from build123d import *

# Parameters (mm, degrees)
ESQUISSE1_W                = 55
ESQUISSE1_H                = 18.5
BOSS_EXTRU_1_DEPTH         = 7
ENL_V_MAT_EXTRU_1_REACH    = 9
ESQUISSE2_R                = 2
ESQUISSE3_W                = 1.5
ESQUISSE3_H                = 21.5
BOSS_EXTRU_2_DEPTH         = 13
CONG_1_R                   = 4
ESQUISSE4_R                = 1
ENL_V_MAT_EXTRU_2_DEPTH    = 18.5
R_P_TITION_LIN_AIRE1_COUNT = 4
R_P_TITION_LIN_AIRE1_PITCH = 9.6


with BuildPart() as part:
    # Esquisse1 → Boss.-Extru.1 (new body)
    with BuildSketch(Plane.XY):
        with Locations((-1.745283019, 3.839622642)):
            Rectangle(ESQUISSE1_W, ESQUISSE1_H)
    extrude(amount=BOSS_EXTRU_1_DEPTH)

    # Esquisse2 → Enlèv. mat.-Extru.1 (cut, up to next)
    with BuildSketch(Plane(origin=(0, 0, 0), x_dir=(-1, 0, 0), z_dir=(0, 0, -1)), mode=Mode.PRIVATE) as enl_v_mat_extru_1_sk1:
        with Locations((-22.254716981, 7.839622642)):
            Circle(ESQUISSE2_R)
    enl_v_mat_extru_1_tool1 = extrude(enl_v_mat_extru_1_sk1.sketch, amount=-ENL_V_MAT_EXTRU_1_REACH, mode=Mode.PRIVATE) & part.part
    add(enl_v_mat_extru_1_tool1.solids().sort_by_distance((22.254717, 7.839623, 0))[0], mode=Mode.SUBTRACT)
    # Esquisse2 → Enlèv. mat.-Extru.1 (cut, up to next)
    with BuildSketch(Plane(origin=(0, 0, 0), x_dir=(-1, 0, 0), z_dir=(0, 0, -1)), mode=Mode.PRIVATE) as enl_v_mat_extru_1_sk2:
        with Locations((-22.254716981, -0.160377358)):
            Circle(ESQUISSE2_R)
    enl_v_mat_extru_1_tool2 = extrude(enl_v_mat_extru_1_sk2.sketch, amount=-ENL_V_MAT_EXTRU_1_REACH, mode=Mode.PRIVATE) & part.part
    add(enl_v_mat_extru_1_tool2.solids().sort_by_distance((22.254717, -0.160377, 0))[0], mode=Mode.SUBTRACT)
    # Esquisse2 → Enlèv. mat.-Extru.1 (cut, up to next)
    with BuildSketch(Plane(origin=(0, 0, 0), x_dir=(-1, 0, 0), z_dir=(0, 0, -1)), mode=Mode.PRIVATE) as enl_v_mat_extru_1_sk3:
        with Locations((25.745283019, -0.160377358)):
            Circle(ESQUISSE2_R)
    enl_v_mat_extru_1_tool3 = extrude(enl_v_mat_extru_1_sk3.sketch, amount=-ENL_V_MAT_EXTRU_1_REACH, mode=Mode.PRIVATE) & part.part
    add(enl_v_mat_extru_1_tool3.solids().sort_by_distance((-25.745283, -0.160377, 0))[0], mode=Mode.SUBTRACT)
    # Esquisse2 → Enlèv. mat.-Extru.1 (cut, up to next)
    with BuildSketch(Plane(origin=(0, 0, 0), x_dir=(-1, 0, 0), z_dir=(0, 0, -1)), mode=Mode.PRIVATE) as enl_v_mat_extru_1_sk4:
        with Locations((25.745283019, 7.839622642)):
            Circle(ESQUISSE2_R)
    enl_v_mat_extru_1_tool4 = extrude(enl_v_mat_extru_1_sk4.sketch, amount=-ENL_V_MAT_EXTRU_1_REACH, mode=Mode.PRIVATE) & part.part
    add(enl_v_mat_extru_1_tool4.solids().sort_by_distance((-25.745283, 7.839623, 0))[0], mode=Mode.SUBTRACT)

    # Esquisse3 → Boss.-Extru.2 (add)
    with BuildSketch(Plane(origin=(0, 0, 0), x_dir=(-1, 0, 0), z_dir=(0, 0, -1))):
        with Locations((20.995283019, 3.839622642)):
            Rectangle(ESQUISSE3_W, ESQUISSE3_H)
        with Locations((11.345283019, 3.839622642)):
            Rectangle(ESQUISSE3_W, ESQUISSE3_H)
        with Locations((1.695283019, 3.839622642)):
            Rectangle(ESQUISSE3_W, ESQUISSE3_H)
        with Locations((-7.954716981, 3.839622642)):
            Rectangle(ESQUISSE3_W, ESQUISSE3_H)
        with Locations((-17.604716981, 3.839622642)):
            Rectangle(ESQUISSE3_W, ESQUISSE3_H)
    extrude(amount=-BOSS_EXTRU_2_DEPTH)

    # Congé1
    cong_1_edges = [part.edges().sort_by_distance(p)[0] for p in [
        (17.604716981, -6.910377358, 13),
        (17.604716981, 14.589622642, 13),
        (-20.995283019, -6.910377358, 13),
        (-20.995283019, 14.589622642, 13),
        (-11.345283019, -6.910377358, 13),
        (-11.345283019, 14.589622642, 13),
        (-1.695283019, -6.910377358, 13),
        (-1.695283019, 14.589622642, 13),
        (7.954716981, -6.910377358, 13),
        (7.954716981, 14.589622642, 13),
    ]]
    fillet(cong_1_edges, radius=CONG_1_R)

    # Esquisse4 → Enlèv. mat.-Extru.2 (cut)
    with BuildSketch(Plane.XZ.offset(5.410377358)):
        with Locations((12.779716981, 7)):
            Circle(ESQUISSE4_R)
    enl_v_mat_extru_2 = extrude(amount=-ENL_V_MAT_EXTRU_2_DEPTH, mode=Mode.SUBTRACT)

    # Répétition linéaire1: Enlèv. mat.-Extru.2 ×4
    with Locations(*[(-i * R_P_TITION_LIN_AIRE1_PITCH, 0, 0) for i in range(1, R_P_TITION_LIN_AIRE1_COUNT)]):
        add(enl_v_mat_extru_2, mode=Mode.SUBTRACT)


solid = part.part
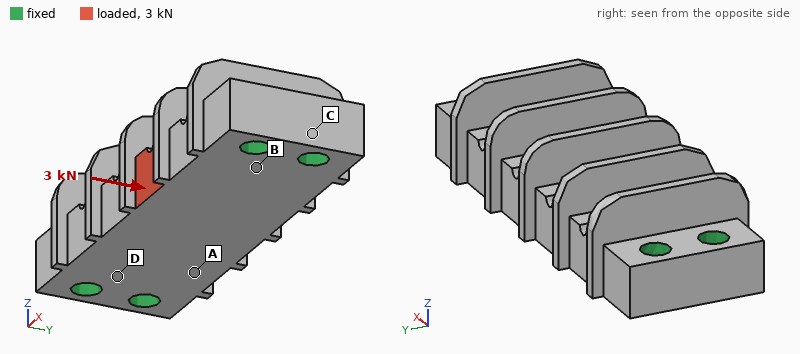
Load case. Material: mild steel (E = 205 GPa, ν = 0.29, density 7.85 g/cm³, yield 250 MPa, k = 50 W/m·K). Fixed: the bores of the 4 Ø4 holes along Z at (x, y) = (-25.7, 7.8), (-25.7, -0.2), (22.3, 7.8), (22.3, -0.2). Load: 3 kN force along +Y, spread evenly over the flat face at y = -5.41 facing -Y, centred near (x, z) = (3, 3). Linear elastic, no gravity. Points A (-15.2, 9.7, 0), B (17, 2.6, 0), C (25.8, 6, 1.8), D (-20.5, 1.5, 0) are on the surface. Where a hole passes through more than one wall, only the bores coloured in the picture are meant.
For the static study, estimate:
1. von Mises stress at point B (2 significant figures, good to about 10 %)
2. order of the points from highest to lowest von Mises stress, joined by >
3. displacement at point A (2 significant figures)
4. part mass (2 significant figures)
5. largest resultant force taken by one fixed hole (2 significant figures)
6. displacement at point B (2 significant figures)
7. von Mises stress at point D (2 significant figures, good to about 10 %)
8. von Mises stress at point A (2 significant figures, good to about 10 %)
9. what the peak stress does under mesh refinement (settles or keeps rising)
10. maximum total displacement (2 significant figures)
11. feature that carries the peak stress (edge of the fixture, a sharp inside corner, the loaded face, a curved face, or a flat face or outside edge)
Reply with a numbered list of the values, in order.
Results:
1. 42 MPa
2. B > D > A > C
3. 2.3 µm
4. 61 g
5. 1.7 kN
6. 1.2 µm
7. 24 MPa
8. 15 MPa
9. keeps rising
10. 7.2 µm
11. a sharp inside corner
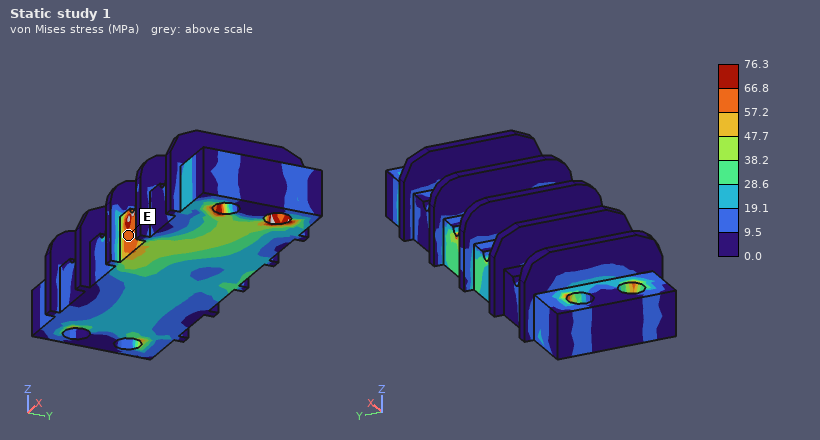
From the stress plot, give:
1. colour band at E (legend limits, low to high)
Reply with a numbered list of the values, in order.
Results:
1. 57.2 to 66.8 MPa
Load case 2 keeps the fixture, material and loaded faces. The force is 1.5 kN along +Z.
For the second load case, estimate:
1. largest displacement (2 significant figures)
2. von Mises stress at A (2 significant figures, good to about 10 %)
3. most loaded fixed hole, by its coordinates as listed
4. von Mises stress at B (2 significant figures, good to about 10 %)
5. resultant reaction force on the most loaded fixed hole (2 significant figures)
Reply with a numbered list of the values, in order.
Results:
1. 19 µm
2. 29 MPa
3. (22.3, -0.2)
4. 55 MPa
5. 1.0 kN
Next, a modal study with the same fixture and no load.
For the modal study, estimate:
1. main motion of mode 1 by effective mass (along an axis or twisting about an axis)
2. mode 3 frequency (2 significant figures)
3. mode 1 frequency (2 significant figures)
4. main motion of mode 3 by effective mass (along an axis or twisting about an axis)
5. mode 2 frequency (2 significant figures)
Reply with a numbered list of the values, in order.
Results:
1. along Z
2. 23 kHz
3. 14 kHz
4. along Y
5. 19 kHz
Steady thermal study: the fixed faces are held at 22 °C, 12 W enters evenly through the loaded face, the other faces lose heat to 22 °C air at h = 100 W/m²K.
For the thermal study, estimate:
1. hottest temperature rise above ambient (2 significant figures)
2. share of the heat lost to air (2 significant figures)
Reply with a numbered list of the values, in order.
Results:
1. 32 K
2. 25 %
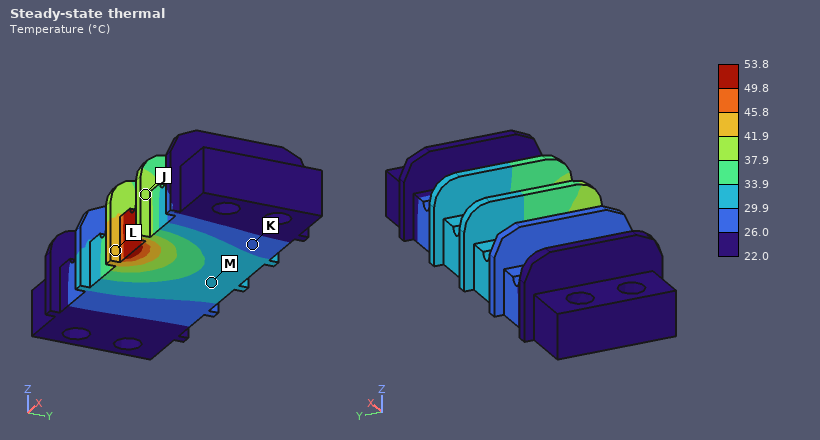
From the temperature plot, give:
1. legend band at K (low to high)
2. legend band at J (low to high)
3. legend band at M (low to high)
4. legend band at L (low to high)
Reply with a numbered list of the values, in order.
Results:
1. 26.0 to 29.9 °C
2. 37.9 to 41.9 °C
3. 29.9 to 33.9 °C
4. 41.9 to 45.8 °C
